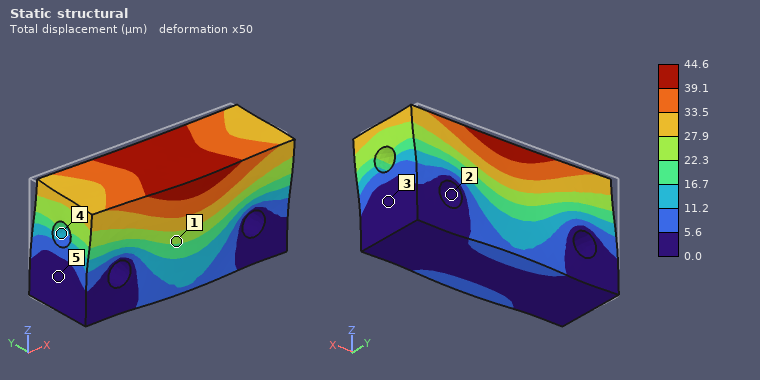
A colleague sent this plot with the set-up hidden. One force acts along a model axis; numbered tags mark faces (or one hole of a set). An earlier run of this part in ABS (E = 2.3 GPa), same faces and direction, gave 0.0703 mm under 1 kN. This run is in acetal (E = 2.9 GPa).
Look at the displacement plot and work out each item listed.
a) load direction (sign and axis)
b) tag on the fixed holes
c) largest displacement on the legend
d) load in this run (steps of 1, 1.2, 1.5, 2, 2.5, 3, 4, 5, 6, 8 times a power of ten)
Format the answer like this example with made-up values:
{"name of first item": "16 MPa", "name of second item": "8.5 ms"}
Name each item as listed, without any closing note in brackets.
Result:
{"load direction": "-Y", "tag on the fixed holes": "2", "largest displacement on the legend": "44.6 µm", "load in this run": "800 N"}
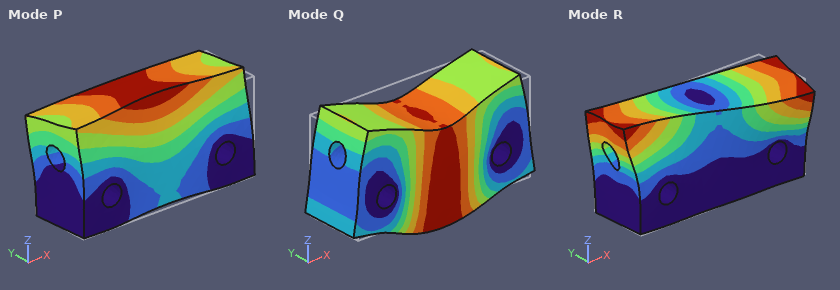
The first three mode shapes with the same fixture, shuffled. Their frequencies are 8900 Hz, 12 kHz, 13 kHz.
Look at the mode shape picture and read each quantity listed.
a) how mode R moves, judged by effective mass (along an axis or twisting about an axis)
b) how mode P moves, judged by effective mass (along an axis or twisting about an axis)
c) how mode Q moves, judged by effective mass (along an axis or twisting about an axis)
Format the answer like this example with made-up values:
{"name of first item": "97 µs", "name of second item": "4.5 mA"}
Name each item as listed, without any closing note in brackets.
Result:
{"how mode R moves, judged by effective mass": "twisting about Z", "how mode P moves, judged by effective mass": "along Y", "how mode Q moves, judged by effective mass": "along Z"}
